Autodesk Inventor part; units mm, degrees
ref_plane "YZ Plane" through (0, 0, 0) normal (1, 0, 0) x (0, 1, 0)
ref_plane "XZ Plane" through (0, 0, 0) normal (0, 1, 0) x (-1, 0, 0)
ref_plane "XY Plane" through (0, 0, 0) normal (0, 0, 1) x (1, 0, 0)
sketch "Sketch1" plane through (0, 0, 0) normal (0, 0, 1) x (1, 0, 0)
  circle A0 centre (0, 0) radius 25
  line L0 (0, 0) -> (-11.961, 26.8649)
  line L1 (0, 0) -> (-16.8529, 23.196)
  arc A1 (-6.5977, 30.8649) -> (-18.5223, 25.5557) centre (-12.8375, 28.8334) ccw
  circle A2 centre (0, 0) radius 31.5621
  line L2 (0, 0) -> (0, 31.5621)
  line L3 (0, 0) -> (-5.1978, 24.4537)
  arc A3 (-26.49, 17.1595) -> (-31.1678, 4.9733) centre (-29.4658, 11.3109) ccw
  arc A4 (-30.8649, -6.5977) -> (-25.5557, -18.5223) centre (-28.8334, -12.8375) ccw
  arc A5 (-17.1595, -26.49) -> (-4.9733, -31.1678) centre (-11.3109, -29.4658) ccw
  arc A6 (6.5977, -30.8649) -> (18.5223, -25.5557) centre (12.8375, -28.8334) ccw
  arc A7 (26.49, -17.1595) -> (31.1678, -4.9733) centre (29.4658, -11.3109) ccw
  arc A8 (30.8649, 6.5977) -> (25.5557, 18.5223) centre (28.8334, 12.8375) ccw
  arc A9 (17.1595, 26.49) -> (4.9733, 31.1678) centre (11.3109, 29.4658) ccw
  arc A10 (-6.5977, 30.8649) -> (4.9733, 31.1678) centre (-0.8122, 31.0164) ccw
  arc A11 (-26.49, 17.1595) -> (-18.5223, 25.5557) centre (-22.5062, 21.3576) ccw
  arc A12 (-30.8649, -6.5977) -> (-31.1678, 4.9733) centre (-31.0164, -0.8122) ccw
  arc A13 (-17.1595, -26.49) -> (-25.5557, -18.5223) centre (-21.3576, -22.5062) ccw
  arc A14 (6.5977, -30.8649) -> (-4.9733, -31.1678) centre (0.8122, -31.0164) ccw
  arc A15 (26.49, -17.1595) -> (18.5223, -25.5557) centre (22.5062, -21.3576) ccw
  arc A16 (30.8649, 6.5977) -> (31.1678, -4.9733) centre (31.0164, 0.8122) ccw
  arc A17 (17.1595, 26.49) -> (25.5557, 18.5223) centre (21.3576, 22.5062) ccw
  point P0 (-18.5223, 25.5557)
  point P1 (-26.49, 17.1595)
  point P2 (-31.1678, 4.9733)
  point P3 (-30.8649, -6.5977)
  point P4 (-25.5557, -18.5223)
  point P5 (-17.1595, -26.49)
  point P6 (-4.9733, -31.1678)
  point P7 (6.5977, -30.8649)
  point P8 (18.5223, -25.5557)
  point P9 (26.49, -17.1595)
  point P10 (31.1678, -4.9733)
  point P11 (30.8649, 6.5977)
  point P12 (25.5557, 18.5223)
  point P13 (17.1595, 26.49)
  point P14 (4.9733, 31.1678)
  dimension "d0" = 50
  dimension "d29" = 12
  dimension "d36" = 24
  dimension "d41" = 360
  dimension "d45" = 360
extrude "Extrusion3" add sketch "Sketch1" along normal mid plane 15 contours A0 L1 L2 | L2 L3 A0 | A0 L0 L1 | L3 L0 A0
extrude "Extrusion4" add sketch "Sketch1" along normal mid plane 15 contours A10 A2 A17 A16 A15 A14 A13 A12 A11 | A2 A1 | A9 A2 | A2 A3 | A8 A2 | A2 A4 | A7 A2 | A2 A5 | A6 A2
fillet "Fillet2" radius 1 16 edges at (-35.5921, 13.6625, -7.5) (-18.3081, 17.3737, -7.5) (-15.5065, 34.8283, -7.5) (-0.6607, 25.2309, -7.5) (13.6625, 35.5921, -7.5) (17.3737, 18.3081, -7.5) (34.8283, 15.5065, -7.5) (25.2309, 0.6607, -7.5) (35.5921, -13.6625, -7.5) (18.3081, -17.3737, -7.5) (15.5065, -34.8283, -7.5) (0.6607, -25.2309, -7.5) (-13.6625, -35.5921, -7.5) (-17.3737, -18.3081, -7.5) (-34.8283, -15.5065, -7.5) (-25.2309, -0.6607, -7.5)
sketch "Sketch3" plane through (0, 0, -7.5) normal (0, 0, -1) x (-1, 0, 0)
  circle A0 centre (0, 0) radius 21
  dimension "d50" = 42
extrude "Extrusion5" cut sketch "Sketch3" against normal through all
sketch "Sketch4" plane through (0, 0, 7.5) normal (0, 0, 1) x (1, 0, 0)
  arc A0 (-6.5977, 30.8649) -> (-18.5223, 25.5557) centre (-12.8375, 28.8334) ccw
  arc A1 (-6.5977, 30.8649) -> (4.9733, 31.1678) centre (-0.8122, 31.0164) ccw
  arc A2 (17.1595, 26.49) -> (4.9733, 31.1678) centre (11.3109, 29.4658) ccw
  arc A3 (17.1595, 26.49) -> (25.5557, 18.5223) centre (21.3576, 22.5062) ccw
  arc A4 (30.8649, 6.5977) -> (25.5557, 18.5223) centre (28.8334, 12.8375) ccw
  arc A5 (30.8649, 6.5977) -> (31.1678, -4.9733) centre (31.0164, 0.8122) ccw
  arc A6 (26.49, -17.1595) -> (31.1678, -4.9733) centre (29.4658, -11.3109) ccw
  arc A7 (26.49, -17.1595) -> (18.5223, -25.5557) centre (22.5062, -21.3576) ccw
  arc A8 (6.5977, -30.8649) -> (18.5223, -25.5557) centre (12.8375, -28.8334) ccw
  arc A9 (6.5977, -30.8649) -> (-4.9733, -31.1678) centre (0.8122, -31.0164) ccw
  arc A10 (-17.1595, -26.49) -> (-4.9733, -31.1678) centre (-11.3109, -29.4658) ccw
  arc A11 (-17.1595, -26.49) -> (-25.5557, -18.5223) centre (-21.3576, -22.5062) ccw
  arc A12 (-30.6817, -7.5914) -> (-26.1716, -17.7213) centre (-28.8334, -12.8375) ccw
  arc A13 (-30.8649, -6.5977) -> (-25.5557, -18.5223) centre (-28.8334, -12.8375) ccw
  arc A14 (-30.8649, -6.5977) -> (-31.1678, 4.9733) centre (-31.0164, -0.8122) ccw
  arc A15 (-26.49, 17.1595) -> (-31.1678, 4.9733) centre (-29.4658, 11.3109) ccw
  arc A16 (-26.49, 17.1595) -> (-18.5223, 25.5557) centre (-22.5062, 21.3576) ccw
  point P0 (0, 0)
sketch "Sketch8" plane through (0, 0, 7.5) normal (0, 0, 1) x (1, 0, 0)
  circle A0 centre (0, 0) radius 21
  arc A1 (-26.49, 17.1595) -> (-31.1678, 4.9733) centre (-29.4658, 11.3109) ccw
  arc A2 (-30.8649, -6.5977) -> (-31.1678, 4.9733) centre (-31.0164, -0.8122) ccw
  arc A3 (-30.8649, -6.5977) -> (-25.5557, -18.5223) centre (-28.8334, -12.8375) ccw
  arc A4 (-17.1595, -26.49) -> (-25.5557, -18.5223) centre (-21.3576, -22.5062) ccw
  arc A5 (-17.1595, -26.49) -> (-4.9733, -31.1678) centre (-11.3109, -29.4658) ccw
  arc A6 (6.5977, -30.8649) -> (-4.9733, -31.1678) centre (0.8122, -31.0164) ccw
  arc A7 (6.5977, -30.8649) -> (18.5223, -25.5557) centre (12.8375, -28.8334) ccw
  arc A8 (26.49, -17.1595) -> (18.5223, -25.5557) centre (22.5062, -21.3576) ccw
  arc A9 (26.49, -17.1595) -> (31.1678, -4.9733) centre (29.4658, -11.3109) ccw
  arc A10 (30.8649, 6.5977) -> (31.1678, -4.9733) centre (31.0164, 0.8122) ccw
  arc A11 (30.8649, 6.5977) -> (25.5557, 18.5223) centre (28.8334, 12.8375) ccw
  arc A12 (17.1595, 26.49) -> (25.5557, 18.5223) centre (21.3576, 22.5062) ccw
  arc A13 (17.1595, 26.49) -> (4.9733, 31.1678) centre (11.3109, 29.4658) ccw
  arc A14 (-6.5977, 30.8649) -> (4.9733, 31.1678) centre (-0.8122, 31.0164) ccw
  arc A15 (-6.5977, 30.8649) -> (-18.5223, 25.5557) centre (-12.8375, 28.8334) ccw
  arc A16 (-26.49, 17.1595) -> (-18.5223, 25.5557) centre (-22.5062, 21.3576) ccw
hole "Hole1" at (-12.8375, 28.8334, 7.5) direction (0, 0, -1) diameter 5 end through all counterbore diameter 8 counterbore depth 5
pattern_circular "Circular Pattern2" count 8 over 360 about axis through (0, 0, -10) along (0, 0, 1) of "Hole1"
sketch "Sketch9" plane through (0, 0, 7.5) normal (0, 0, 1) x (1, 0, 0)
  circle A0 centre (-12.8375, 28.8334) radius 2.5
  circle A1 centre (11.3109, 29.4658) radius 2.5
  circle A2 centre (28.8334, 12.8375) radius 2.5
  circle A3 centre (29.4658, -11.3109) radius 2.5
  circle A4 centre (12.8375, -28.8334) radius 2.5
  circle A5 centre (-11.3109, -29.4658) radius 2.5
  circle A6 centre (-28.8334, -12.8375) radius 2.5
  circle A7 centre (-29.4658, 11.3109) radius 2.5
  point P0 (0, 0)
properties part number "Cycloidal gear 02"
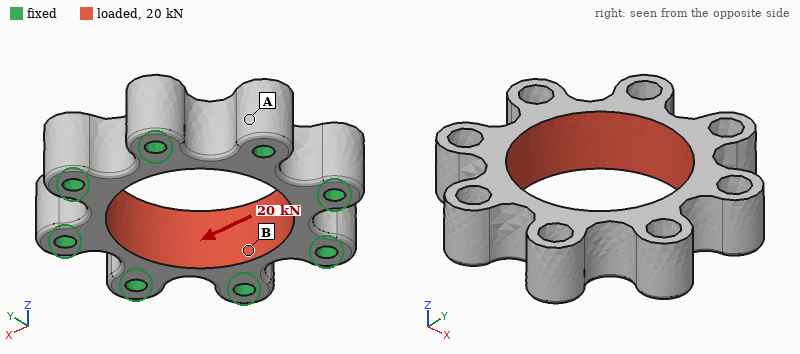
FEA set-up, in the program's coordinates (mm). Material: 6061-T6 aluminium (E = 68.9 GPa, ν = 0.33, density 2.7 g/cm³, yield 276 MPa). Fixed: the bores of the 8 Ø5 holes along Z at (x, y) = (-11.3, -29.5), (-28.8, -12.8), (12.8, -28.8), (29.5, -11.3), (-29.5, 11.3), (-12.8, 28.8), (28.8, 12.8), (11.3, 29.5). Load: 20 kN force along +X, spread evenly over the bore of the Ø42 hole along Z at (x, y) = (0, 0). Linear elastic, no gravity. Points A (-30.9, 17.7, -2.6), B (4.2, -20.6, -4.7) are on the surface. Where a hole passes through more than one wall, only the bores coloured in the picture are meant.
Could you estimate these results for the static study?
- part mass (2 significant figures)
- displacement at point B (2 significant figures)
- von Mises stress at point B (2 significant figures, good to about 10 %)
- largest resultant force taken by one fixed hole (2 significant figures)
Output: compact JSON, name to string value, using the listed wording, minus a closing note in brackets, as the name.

{"part mass": "65 g", "displacement at point B": "4.2 µm", "von Mises stress at point B": "21 MPa", "largest resultant force taken by one fixed hole": "3.3 kN"}
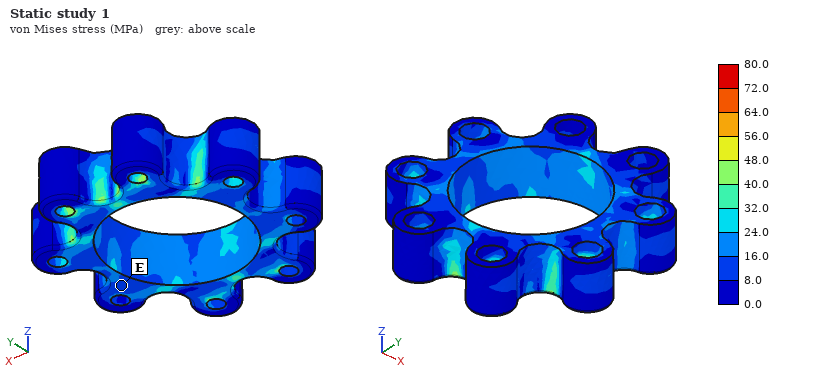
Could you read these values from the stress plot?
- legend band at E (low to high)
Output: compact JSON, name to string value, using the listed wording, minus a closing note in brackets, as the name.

{"legend band at E": "8.0 to 16.0 MPa"}
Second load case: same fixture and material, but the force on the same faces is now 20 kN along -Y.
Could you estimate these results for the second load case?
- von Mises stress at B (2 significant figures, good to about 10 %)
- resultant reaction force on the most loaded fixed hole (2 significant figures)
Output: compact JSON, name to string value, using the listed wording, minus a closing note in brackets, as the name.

{"von Mises stress at B": "12 MPa", "resultant reaction force on the most loaded fixed hole": "3.3 kN"}
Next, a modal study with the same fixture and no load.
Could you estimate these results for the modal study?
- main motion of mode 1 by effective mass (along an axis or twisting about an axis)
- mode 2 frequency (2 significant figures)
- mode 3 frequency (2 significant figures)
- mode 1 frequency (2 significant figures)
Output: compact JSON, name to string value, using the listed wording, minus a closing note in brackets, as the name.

{"main motion of mode 1 by effective mass": "along Z", "mode 2 frequency": "40 kHz", "mode 3 frequency": "40 kHz", "mode 1 frequency": "38 kHz"}
